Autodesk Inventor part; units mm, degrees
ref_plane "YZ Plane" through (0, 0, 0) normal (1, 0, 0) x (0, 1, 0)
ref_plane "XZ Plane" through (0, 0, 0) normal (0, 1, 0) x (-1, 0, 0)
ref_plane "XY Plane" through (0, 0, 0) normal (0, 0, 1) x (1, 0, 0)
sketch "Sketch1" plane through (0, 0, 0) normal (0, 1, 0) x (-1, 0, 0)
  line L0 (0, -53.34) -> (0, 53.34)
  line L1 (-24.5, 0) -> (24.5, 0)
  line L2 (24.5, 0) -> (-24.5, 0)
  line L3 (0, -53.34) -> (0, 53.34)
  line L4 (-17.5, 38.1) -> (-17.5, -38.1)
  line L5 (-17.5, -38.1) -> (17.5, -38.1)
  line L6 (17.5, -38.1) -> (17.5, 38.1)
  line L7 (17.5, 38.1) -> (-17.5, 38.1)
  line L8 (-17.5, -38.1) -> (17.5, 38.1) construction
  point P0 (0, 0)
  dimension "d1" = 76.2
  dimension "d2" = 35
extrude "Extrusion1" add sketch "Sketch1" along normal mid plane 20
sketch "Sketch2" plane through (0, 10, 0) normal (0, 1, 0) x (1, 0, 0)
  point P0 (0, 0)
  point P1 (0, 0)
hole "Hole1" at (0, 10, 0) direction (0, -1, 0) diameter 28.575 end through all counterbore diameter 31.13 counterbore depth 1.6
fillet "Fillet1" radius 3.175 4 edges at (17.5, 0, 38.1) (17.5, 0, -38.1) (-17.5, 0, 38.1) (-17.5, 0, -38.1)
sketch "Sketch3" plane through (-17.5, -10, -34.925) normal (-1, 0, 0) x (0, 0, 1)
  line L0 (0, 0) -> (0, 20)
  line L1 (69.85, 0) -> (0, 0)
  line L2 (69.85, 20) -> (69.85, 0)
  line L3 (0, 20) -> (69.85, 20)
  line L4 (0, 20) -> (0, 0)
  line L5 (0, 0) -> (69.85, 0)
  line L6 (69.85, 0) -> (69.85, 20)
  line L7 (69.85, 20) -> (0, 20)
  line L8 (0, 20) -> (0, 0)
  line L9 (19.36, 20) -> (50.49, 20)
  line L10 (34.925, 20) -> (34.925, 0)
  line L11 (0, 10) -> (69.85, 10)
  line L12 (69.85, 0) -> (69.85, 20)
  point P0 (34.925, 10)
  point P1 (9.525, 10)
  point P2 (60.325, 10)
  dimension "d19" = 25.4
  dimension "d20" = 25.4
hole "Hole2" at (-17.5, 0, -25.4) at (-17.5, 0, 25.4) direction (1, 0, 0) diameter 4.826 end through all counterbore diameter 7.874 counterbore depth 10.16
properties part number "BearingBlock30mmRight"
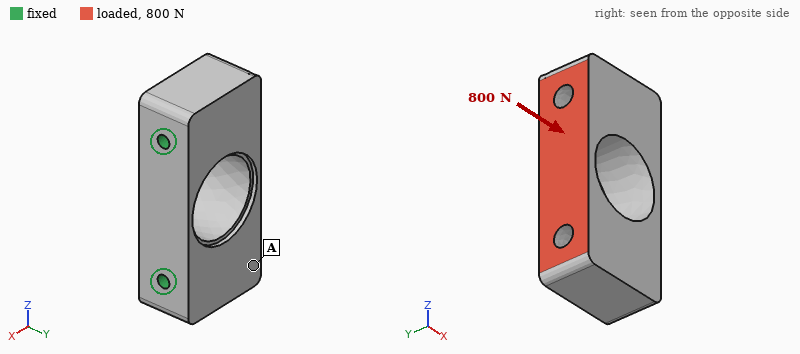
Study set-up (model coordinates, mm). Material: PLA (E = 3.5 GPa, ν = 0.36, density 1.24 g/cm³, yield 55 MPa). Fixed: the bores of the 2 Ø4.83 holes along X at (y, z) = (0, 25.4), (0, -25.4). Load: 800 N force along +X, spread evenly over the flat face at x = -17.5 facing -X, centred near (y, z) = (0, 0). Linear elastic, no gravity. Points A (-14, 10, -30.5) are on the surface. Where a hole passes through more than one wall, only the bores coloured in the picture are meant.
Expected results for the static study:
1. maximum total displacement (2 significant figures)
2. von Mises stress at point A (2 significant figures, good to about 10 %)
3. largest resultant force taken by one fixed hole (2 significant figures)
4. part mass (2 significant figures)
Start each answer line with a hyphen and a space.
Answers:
- 39 µm
- 0.71 MPa
- 420 N
- 47 g
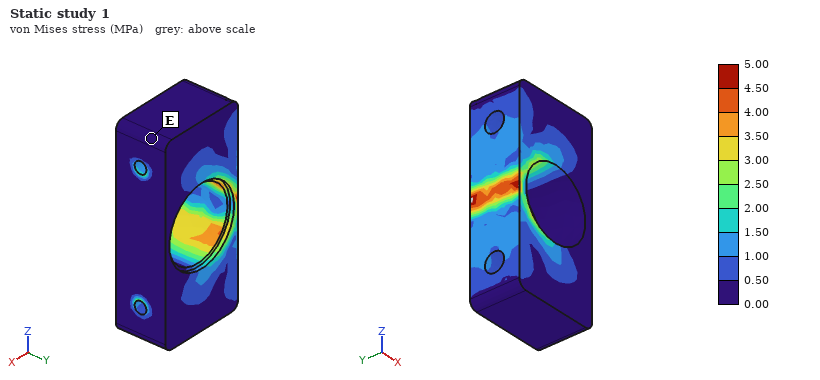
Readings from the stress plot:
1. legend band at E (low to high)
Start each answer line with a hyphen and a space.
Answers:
- 0.00 to 0.50 MPa
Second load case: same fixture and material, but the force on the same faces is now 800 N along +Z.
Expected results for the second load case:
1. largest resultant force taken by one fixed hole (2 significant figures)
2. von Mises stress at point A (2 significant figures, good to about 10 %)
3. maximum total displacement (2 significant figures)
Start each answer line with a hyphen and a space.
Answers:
- 410 N
- 1.3 MPa
- 34 µm
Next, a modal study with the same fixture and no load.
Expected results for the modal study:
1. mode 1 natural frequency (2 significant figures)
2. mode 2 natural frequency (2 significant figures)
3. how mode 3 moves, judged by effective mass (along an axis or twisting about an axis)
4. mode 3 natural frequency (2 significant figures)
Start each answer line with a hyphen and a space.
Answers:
- 5300 Hz
- 7000 Hz
- along Z
- 7600 Hz
